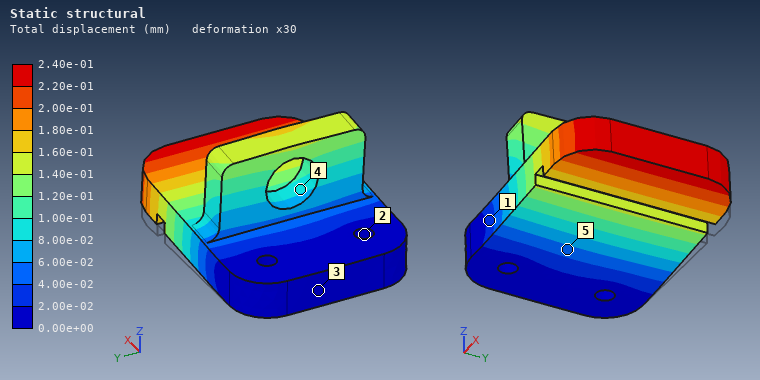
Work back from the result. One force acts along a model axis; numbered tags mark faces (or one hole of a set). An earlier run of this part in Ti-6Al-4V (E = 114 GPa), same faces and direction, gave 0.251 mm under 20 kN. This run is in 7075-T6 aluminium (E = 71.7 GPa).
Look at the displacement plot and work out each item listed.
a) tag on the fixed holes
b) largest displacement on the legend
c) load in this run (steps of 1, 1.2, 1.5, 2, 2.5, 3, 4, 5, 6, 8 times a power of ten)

2
2.40e-01 mm
12 kN
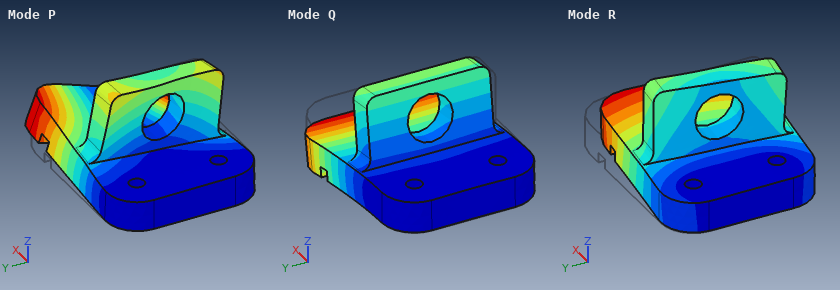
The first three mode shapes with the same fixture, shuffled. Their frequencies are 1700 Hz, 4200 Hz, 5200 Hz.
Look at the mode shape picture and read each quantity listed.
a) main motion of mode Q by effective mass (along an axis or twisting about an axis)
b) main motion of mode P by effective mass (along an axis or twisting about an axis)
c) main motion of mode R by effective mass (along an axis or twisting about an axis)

along Z
twisting about X
along Y
